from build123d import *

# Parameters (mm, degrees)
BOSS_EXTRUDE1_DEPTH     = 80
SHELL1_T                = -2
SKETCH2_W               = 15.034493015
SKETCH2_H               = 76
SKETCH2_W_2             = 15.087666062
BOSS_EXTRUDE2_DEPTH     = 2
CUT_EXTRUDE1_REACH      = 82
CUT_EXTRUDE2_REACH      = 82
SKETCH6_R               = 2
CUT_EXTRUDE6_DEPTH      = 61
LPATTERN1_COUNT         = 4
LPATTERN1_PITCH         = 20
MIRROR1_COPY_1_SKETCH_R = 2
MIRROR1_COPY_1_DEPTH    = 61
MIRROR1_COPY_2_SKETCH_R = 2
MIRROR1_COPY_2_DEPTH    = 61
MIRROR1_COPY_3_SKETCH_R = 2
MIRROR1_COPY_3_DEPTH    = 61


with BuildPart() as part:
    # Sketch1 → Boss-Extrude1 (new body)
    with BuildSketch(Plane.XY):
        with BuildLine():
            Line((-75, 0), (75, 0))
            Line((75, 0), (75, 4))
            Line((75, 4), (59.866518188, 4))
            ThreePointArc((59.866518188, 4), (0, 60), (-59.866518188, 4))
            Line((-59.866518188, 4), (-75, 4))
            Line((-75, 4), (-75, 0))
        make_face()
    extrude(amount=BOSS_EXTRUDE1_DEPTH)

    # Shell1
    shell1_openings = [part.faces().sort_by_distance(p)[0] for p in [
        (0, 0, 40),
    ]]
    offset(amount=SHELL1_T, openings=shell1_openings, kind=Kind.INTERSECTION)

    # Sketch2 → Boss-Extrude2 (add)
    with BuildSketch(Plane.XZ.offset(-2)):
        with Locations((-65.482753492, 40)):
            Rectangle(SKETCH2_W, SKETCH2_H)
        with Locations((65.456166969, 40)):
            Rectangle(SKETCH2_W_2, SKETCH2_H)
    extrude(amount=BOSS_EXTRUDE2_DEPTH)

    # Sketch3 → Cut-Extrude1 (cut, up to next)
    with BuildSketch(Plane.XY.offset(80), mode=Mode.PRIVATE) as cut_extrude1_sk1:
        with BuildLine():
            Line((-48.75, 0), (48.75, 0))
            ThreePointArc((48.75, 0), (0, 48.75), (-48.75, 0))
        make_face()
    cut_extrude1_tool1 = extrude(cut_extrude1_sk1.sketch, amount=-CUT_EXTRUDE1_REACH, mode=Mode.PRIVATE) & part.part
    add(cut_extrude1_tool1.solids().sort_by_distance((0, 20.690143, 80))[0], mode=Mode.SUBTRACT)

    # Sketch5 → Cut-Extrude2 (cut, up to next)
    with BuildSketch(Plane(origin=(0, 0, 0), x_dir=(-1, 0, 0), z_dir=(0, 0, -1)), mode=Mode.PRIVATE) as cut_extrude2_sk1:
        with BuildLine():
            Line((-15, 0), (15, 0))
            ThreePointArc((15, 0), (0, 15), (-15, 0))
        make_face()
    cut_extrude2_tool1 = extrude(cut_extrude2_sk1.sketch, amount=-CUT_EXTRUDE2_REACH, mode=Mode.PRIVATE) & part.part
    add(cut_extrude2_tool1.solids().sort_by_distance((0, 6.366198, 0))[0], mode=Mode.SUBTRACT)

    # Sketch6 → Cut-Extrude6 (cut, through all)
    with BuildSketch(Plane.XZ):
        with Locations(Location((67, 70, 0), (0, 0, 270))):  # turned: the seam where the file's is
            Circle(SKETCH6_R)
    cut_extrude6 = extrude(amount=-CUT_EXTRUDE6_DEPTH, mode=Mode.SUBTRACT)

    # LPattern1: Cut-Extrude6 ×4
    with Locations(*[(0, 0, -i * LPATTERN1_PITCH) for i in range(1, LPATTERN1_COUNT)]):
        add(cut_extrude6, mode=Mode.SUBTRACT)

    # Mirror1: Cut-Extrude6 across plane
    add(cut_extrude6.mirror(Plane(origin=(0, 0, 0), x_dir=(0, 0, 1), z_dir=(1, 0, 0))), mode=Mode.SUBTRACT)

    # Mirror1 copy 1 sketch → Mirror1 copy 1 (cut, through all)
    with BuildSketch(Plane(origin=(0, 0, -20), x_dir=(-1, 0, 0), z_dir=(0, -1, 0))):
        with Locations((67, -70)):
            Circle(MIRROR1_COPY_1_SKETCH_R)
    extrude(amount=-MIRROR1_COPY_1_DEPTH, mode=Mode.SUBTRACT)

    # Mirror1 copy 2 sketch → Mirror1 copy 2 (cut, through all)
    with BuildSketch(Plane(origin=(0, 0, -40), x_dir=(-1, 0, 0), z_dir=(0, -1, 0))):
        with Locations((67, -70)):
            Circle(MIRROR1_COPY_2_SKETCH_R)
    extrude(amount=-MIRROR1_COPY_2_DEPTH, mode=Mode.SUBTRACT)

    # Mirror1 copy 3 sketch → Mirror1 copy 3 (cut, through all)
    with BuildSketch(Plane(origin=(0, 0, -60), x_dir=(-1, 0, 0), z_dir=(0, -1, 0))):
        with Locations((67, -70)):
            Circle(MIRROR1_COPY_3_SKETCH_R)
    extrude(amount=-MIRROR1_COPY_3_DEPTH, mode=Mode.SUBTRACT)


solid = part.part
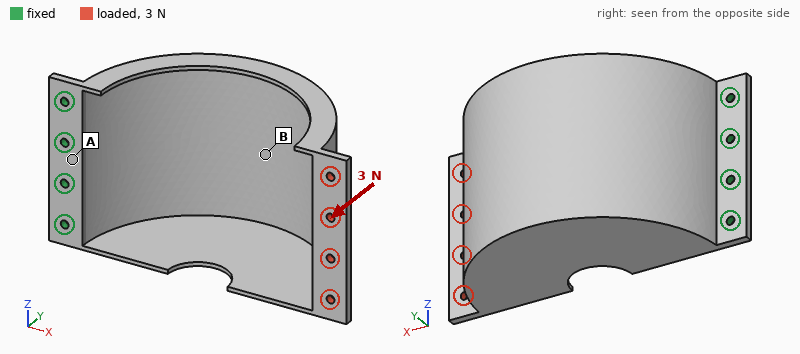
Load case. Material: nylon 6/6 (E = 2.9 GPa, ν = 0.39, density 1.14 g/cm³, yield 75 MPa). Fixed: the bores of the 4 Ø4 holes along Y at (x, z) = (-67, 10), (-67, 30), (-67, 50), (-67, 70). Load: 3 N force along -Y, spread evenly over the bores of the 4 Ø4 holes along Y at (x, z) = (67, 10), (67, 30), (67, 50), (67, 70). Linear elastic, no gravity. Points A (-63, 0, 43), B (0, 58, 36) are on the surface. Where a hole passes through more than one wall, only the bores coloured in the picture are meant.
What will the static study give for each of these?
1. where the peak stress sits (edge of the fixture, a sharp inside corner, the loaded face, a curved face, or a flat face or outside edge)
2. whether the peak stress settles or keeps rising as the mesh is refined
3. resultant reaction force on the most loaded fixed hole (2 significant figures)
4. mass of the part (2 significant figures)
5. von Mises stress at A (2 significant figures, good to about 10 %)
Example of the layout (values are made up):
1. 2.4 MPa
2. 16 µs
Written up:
1. a sharp inside corner
2. keeps rising
3. 8.9 N
4. 59 g
5. 0.61 MPa
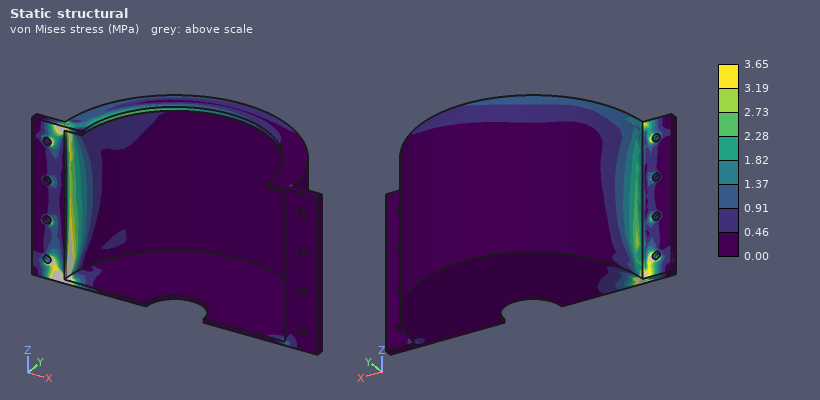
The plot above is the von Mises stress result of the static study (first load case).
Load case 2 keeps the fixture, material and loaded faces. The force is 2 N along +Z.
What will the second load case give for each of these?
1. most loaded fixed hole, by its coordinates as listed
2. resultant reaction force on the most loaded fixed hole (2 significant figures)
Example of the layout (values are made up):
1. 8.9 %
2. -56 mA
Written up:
1. (-67, 10)
2. 5.3 N
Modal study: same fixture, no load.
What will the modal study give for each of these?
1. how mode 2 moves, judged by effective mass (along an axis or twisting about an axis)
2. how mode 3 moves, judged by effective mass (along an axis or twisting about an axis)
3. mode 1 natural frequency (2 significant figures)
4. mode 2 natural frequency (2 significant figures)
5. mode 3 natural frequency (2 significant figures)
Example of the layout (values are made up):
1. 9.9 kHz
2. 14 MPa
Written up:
1. along Y
2. along X
3. 40 Hz
4. 45 Hz
5. 170 Hz
